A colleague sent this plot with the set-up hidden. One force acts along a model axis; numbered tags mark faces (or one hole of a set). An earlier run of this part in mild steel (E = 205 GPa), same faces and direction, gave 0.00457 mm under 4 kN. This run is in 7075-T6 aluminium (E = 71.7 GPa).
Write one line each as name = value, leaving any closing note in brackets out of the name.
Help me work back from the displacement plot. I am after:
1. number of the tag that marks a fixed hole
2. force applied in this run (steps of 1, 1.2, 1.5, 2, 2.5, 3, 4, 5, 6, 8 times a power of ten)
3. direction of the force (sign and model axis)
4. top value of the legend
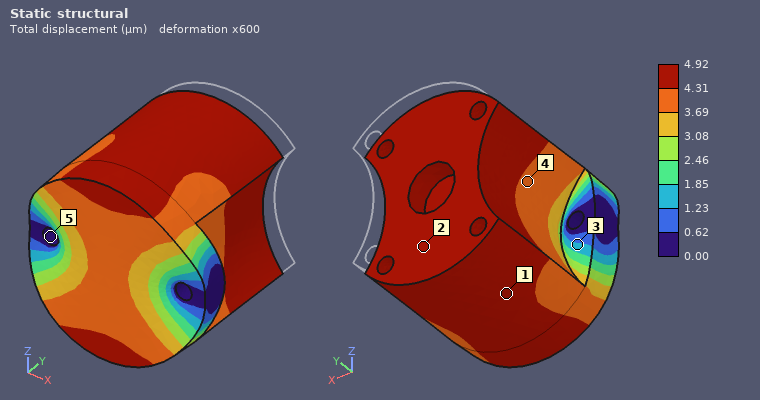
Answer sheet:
number of the tag that marks a fixed hole = 5
force applied in this run = 1.5 kN
direction of the force = -Y
top value of the legend = 4.92 µm
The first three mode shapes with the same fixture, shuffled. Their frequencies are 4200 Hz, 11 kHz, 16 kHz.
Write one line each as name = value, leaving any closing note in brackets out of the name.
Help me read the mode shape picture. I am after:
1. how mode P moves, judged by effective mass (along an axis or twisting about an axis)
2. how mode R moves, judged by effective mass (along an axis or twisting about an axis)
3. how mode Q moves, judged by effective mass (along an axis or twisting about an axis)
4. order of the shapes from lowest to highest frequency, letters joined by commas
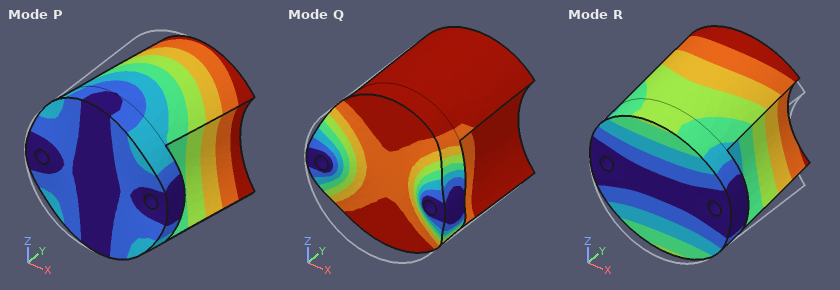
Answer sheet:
how mode P moves, judged by effective mass = along X
how mode R moves, judged by effective mass = along Z
how mode Q moves, judged by effective mass = along Y
order of the shapes from lowest to highest frequency, letters joined by commas = R, P, Q
